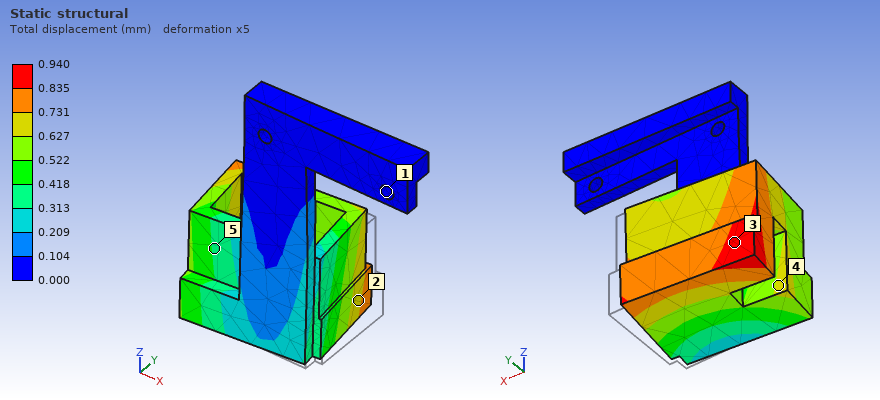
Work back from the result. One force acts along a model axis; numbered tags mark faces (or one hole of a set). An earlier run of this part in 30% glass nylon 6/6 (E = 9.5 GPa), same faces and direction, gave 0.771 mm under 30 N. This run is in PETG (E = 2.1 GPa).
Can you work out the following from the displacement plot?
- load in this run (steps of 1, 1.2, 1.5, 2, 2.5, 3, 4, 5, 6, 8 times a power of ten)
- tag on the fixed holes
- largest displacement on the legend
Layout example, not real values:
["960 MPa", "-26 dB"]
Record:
["8 N", "1", "0.940 mm"]
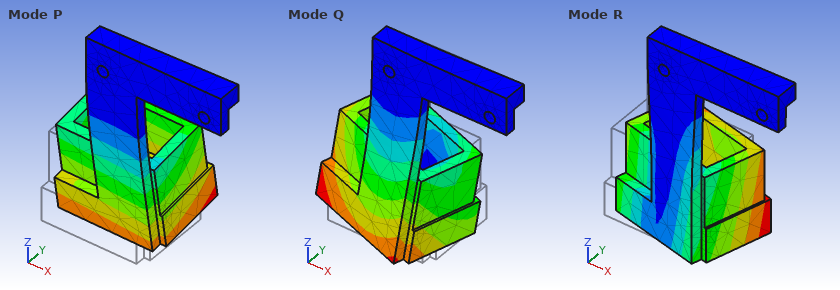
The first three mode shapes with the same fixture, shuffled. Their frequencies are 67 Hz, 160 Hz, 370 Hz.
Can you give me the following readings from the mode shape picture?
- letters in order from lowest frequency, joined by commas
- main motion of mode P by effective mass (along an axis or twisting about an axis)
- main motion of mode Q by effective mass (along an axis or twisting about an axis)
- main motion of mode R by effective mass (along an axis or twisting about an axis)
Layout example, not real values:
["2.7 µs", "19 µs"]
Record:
["P, R, Q", "along Y", "along X", "along X"]
